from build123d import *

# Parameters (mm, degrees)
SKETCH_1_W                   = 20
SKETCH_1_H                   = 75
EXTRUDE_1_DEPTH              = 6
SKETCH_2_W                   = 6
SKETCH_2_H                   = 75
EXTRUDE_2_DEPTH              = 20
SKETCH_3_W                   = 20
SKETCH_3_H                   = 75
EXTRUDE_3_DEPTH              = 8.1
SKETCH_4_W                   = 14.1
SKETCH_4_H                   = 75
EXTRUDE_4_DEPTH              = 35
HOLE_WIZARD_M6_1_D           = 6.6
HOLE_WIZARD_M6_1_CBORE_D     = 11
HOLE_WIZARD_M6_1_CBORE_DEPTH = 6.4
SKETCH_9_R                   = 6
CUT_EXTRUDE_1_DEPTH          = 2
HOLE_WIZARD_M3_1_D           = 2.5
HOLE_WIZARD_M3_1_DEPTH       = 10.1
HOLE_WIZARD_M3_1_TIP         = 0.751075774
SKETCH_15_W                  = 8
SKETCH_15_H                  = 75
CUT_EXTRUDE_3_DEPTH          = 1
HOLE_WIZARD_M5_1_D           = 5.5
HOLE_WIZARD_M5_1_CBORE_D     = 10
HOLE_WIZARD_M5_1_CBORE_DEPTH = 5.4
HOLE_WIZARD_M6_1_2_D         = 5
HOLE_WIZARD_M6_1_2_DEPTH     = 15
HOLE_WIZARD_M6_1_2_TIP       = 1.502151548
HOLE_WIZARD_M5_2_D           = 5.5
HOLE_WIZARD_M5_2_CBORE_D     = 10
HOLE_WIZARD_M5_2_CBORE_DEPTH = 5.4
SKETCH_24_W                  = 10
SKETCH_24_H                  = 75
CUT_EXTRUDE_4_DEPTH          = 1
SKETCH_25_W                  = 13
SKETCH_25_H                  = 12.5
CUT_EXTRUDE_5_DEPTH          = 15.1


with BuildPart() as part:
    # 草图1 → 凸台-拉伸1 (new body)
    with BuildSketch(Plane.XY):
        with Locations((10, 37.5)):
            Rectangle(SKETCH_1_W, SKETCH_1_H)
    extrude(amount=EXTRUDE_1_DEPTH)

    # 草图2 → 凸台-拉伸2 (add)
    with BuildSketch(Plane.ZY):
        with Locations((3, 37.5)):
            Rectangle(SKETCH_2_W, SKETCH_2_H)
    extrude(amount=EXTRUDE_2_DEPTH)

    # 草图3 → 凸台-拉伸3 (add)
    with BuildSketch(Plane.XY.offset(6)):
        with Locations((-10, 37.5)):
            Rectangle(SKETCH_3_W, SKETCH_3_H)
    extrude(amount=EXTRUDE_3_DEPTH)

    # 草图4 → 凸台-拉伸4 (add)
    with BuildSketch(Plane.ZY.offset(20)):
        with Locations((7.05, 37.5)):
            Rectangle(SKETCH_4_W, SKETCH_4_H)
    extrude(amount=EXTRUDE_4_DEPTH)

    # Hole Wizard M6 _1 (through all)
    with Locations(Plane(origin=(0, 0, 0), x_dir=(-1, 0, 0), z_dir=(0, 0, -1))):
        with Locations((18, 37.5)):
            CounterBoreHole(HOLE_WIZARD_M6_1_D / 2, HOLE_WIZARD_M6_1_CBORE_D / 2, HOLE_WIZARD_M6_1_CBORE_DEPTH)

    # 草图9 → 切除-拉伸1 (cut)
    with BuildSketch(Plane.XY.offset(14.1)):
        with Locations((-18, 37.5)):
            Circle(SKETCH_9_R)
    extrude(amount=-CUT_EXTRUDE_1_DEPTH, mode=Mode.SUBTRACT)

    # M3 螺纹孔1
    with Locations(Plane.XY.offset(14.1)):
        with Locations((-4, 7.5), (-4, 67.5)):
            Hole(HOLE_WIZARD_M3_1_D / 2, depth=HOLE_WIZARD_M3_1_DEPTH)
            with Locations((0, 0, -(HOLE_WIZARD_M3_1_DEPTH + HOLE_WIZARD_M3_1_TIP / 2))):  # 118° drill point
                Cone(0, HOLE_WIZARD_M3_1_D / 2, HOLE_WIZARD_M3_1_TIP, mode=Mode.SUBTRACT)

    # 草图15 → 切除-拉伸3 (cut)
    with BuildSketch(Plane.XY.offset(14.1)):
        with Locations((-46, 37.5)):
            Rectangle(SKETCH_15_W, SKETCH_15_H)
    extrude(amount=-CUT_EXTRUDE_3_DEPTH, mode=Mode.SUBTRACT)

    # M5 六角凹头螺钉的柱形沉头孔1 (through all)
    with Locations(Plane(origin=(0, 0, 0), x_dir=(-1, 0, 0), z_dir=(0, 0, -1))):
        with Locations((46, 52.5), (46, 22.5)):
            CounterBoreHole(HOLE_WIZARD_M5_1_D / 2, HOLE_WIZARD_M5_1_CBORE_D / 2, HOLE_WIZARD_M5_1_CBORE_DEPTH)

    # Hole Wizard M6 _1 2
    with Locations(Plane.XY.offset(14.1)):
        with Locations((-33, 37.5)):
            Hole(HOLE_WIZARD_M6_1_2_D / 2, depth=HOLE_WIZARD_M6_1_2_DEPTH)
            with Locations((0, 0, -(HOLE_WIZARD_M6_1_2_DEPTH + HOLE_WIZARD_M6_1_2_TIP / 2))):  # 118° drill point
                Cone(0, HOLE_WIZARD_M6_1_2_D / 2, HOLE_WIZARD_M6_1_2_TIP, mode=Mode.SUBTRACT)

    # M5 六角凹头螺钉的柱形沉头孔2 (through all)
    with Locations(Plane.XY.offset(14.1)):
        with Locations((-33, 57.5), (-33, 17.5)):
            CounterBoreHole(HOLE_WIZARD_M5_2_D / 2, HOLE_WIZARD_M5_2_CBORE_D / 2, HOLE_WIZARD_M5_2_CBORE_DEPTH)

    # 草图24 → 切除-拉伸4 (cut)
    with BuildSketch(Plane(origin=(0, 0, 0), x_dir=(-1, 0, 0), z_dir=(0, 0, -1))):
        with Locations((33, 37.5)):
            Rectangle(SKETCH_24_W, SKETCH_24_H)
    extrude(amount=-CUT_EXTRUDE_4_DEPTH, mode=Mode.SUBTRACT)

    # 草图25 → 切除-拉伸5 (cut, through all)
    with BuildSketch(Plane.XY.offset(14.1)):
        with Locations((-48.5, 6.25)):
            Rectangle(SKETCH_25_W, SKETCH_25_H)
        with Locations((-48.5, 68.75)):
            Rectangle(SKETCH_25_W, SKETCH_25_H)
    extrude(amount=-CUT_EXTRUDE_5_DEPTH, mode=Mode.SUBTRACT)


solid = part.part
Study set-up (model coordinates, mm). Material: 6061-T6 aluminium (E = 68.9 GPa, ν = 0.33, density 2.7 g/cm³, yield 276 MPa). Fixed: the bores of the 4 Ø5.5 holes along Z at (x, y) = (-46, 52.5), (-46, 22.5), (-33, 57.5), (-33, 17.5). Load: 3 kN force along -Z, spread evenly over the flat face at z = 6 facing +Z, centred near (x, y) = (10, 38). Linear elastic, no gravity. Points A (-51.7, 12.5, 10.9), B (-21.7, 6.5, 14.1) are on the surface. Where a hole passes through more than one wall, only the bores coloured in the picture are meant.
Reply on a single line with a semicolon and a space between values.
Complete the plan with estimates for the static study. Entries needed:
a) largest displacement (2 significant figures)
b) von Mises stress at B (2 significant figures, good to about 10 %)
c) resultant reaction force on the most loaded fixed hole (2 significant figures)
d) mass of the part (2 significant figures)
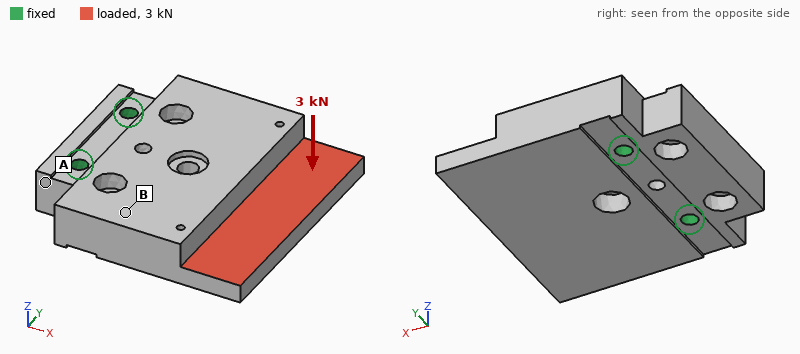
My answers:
0.24 mm; 40 MPa; 3.9 kN; 160 g
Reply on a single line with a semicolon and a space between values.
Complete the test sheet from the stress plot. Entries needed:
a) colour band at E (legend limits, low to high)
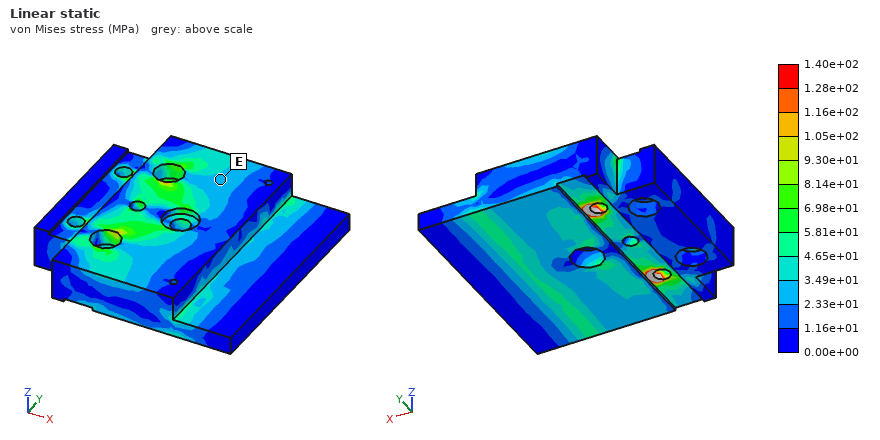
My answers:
2.33e+01 to 3.49e+01 MPa
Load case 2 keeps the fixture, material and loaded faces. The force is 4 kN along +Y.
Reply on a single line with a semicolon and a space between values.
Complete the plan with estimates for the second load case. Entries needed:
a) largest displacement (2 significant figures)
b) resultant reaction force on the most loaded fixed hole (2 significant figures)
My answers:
37 µm; 3.9 kN
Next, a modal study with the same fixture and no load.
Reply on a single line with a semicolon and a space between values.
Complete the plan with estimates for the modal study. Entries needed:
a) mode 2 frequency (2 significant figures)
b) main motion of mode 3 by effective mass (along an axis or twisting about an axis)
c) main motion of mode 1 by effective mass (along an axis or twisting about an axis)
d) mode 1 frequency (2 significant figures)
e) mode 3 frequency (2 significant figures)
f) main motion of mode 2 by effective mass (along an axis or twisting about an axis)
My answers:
5700 Hz; along Y; along Z; 3500 Hz; 9400 Hz; twisting about X
